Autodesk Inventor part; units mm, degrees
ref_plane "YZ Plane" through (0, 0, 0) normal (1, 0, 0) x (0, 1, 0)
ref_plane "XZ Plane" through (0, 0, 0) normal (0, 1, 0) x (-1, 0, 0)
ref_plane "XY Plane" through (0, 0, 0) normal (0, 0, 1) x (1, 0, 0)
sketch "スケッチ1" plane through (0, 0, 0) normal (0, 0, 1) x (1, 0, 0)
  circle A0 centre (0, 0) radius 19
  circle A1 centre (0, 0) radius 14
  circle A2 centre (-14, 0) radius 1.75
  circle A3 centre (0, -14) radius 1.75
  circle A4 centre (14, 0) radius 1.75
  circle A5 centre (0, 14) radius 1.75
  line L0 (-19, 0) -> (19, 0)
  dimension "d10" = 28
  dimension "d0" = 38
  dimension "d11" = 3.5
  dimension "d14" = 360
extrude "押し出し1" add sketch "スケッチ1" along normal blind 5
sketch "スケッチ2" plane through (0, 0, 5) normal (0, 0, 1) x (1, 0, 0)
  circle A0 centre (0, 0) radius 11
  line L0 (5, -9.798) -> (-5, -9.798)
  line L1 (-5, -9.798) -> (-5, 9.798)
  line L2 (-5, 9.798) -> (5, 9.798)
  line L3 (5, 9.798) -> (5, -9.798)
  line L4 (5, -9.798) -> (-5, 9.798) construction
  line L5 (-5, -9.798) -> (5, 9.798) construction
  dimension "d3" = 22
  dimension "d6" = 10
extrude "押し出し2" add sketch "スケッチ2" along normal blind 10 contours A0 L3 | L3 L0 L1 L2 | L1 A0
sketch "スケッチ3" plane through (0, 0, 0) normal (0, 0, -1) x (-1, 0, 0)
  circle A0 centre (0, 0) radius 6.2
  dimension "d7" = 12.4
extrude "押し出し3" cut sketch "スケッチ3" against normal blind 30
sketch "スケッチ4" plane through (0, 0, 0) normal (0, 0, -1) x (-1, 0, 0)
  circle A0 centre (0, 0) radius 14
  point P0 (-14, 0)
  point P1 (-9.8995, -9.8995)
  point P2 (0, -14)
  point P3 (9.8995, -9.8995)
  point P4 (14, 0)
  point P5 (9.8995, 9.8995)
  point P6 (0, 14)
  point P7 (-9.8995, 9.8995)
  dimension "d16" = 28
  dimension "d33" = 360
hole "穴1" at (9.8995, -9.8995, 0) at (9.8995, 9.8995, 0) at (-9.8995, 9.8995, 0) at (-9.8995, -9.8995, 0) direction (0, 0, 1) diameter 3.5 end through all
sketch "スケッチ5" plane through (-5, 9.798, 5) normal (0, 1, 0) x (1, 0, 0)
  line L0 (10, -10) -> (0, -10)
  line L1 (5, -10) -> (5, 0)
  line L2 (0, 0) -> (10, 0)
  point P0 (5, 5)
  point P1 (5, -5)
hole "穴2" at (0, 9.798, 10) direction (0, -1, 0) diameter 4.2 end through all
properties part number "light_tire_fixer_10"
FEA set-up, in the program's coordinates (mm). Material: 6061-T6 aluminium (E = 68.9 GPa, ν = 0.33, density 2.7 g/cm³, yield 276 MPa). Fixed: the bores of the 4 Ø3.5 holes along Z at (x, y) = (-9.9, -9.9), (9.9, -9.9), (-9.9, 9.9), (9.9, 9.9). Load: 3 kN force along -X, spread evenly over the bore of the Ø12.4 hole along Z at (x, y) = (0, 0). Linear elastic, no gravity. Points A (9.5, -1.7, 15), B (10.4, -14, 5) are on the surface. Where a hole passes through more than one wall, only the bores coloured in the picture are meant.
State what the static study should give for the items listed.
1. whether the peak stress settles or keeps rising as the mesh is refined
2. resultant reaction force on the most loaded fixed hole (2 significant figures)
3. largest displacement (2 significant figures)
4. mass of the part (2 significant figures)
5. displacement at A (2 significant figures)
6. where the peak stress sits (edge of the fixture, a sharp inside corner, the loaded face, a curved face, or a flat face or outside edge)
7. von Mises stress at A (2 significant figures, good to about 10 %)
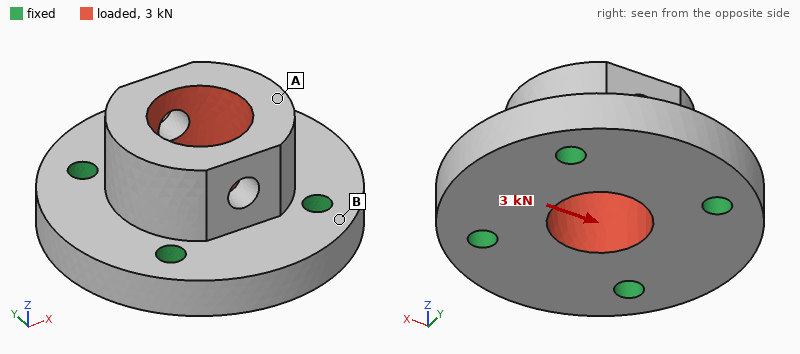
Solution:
keeps rising
840 N
9.1 µm
19 g
8.9 µm
edge of the fixture
12 MPa
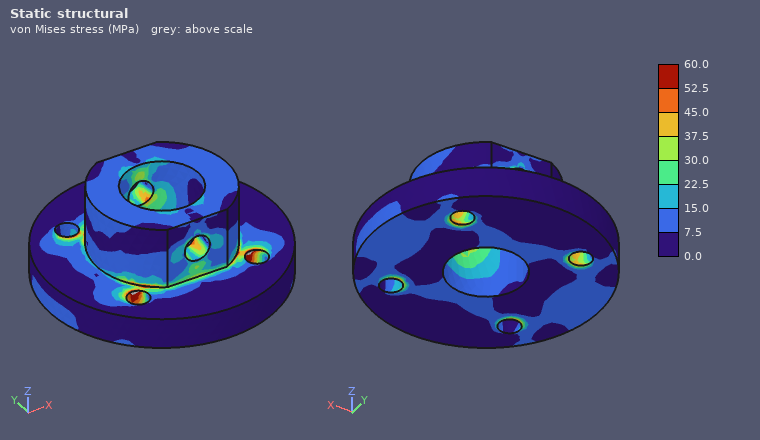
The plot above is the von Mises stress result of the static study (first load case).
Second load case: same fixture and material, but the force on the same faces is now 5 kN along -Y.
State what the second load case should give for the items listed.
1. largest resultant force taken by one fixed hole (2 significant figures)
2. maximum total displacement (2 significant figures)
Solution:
1.4 kN
14 µm
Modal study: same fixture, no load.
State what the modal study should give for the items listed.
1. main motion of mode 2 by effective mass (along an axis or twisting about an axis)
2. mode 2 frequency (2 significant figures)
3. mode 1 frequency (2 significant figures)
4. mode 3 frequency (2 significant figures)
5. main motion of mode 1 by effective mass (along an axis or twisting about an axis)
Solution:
along Y
35 kHz
33 kHz
38 kHz
along X
